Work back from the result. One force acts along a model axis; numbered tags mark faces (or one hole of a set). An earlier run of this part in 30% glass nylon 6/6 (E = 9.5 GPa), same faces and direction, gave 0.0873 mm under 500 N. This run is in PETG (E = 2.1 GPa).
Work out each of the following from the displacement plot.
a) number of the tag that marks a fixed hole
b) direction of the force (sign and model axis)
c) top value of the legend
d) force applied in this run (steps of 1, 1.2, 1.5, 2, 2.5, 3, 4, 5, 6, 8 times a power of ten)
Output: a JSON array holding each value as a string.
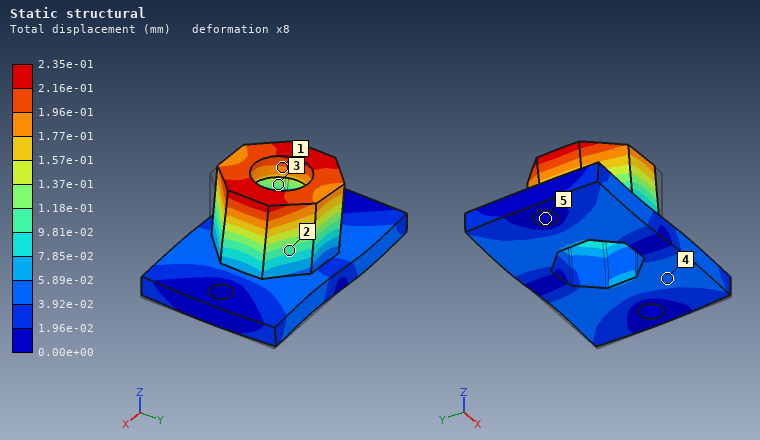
["5", "-X", "2.35e-01 mm", "300 N"]
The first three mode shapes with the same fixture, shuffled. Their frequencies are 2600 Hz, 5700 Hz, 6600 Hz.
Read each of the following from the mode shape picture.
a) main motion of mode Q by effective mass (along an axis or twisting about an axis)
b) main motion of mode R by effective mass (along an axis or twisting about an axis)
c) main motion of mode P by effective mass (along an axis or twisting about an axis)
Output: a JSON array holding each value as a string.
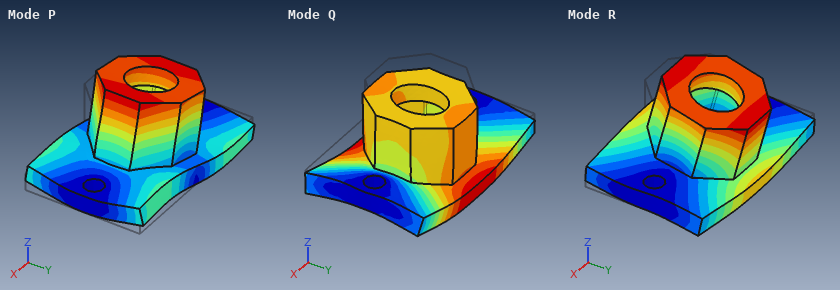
["along Z", "along Y", "along X"]
